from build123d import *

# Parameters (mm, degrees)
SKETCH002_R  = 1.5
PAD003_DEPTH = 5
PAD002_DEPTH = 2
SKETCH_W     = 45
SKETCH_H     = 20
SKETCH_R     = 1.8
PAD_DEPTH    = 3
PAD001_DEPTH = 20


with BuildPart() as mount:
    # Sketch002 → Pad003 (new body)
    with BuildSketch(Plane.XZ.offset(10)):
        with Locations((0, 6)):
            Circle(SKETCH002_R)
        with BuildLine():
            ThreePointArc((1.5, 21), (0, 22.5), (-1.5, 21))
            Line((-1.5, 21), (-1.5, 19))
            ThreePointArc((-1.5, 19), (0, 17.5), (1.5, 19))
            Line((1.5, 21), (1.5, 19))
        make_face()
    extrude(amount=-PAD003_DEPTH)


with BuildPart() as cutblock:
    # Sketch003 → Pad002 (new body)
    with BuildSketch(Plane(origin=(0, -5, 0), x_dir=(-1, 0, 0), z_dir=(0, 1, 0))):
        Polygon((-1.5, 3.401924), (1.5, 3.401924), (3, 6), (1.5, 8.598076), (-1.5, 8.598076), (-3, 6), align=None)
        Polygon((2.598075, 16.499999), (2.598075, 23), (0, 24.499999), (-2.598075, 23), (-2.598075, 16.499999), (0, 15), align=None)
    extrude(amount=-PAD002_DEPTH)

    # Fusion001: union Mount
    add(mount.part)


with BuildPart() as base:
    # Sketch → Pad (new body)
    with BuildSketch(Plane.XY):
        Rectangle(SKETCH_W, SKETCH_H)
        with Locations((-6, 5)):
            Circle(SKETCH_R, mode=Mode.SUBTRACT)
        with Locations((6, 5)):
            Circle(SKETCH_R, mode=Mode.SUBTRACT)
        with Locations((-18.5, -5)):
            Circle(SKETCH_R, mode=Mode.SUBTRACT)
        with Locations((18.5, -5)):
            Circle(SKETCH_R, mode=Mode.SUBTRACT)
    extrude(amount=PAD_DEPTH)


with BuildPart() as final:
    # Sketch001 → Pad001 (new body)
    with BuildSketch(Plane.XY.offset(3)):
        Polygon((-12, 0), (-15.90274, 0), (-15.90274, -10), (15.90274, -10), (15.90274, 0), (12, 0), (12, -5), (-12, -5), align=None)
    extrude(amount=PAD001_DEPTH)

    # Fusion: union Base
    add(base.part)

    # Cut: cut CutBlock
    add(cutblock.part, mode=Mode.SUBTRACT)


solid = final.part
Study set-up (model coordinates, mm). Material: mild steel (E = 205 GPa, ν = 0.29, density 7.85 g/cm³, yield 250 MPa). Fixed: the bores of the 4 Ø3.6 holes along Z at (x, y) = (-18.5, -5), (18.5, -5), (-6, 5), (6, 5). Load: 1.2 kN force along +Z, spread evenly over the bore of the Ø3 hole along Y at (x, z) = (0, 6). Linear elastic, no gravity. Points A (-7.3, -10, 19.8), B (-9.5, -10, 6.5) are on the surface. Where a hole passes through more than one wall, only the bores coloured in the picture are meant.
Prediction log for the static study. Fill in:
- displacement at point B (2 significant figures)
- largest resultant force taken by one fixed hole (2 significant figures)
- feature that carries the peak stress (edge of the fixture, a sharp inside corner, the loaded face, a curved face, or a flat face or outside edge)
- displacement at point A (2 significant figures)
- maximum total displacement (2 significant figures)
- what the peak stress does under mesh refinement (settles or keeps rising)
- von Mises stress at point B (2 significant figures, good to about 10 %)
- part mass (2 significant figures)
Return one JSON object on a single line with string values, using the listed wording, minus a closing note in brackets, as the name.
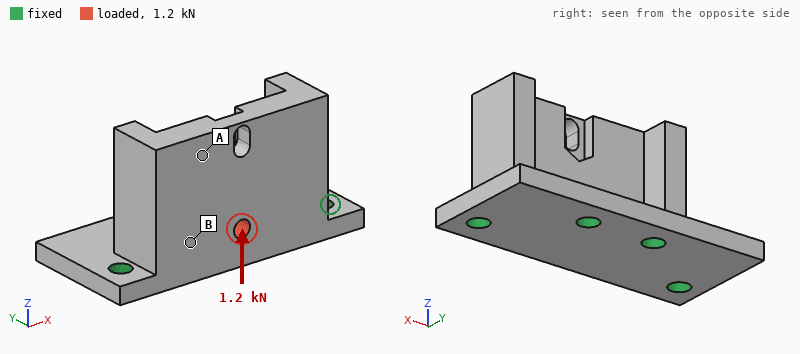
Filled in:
{"displacement at point B": "5.9 µm", "largest resultant force taken by one fixed hole": "710 N", "feature that carries the peak stress": "edge of the fixture", "displacement at point A": "12 µm", "maximum total displacement": "15 µm", "what the peak stress does under mesh refinement": "keeps rising", "von Mises stress at point B": "23 MPa", "part mass": "50 g"}
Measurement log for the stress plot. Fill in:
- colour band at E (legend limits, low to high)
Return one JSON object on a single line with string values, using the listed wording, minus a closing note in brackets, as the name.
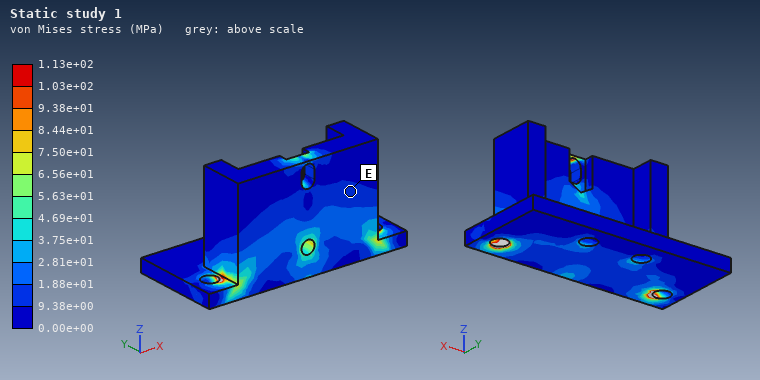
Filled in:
{"colour band at E": "9.38e+00 to 1.88e+01 MPa"}
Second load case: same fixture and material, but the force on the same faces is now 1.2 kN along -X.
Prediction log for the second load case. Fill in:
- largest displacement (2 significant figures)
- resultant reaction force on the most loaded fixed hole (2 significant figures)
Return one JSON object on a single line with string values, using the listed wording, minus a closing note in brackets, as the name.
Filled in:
{"largest displacement": "1.8 µm", "resultant reaction force on the most loaded fixed hole": "500 N"}
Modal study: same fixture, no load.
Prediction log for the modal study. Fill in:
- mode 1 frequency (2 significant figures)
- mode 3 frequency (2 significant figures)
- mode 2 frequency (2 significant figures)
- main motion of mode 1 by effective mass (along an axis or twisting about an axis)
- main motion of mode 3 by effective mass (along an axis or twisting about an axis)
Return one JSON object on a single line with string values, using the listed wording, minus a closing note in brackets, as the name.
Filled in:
{"mode 1 frequency": "6700 Hz", "mode 3 frequency": "21 kHz", "mode 2 frequency": "12 kHz", "main motion of mode 1 by effective mass": "along Y", "main motion of mode 3 by effective mass": "along X"}
